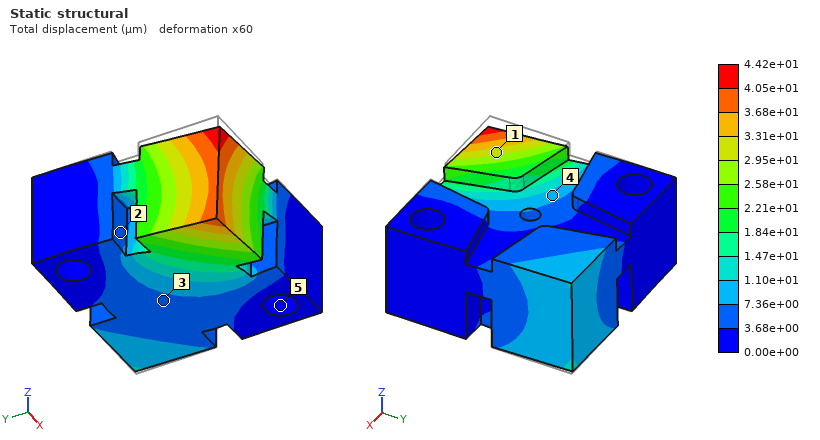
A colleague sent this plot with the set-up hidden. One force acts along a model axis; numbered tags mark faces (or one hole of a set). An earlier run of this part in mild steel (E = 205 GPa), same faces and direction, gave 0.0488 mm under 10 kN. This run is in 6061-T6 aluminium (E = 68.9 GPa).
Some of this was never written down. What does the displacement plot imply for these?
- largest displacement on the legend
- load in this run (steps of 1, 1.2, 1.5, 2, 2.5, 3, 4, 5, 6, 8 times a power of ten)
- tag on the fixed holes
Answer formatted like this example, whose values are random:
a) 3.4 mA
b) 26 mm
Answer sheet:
a) 4.42e+01 µm
b) 3 kN
c) 5
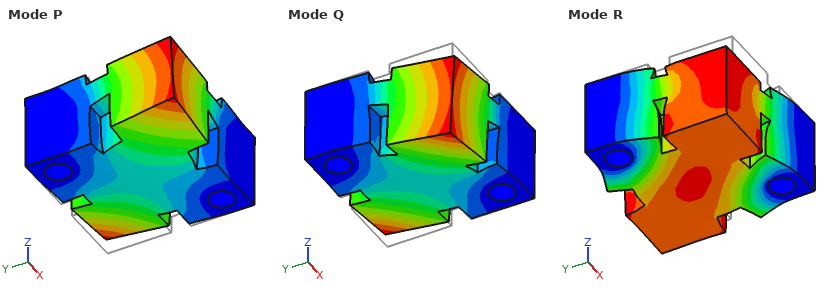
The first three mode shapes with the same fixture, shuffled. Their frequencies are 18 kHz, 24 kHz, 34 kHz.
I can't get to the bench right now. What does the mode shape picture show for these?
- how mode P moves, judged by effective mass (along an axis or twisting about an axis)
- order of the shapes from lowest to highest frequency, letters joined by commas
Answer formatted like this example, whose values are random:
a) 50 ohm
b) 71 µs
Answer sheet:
a) along Z
b) Q, P, R
